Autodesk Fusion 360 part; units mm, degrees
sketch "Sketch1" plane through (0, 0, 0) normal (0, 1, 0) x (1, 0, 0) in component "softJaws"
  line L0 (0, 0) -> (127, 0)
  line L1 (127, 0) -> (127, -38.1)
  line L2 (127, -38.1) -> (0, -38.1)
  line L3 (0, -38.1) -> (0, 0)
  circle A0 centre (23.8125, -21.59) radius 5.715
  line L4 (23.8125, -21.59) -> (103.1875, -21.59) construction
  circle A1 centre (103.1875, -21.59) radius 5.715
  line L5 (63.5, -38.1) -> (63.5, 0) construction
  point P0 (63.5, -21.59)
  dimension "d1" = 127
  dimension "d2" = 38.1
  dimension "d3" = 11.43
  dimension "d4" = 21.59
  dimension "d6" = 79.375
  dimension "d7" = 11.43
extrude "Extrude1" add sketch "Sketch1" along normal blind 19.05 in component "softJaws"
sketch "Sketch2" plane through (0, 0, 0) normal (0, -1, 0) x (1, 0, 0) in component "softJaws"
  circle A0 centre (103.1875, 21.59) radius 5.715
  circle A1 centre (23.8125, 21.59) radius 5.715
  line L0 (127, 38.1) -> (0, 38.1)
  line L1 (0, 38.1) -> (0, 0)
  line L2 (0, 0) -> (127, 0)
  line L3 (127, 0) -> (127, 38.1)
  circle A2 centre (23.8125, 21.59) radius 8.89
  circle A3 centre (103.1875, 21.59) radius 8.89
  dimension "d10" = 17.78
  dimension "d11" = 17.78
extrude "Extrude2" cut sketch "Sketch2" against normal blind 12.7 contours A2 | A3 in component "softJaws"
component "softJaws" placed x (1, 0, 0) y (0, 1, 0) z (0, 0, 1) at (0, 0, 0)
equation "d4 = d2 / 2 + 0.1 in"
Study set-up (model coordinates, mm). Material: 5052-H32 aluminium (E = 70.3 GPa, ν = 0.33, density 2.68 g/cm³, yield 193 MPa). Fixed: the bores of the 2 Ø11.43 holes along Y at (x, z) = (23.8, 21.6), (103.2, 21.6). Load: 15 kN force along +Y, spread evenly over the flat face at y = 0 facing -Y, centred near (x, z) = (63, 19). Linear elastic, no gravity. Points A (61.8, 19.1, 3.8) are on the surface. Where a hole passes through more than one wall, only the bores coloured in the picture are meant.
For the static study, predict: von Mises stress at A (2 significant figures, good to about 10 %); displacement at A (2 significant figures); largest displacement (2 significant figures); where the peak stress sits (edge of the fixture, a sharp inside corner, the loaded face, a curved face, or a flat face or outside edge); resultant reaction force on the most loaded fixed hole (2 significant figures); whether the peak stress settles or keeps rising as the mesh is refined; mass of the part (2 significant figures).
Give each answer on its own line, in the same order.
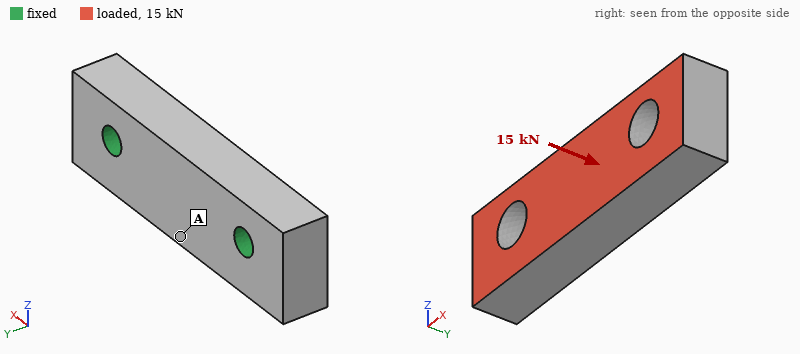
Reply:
16 MPa
33 µm
38 µm
edge of the fixture
7.8 kN
keeps rising
230 g
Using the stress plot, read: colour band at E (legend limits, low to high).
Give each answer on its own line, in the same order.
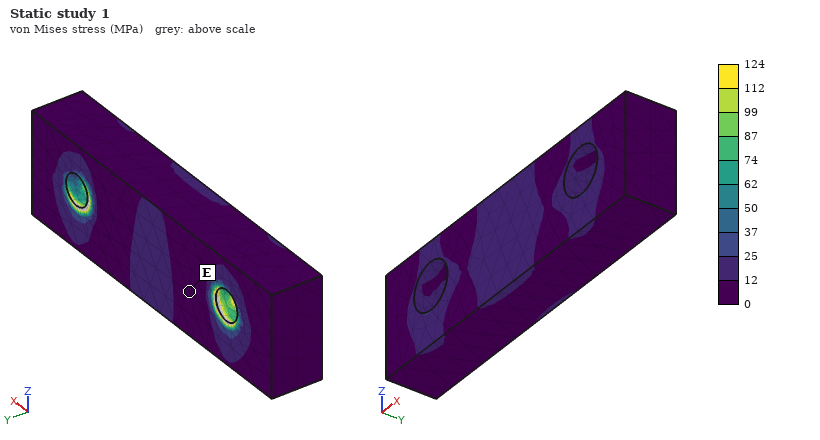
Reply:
0 to 12 MPa
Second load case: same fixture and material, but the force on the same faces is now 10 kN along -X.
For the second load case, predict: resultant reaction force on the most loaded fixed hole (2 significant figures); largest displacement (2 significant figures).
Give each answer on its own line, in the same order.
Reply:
5.3 kN
19 µm
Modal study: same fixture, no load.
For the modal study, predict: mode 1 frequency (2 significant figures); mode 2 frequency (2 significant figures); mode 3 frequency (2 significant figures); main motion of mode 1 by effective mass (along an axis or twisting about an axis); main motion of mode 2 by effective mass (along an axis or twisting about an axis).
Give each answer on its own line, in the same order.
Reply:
6100 Hz
8600 Hz
10000 Hz
along Z
along Y
